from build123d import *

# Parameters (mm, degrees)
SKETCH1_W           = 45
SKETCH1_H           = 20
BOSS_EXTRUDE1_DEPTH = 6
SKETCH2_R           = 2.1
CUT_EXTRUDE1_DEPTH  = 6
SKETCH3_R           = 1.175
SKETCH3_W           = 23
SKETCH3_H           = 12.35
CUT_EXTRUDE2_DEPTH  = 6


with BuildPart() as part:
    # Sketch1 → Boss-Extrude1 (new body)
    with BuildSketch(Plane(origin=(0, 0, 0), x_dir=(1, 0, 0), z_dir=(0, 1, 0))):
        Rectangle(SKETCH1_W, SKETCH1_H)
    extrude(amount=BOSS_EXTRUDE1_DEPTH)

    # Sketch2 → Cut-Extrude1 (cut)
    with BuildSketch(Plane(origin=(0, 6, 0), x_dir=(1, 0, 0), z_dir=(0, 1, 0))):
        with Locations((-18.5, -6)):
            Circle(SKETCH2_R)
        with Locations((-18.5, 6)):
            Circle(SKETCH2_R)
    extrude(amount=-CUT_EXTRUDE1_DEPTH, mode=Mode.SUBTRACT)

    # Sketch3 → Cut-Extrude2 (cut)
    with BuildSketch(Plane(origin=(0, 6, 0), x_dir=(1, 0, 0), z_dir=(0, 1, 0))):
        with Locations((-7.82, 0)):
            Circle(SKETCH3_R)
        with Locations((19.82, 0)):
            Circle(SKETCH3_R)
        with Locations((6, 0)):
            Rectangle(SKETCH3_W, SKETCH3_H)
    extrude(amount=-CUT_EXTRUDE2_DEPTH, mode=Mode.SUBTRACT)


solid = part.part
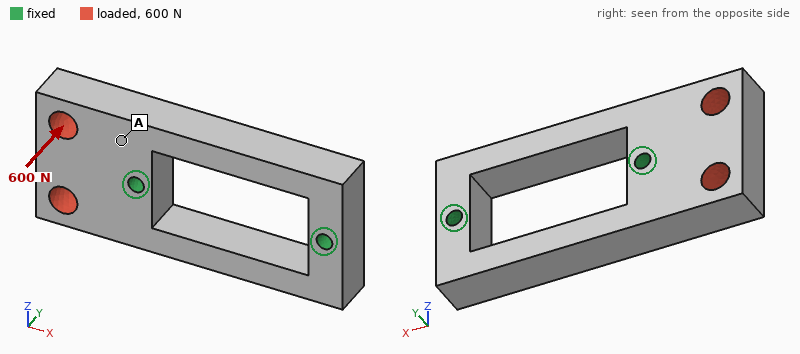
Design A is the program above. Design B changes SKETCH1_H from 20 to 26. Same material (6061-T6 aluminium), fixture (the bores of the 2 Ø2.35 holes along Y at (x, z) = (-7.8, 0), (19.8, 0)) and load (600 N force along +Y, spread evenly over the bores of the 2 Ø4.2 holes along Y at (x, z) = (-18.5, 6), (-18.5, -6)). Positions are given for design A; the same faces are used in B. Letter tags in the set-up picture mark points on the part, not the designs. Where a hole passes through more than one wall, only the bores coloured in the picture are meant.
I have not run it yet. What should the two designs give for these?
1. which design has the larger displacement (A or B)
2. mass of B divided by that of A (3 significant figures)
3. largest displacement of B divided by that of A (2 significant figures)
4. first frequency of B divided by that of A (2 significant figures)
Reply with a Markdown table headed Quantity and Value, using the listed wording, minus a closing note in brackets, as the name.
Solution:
| Quantity | Value |
|---|---|
| which design has the larger displacement | A |
| mass of B divided by that of A | 1.47 |
| largest displacement of B divided by that of A | 0.86 |
| first frequency of B divided by that of A | 0.86 |
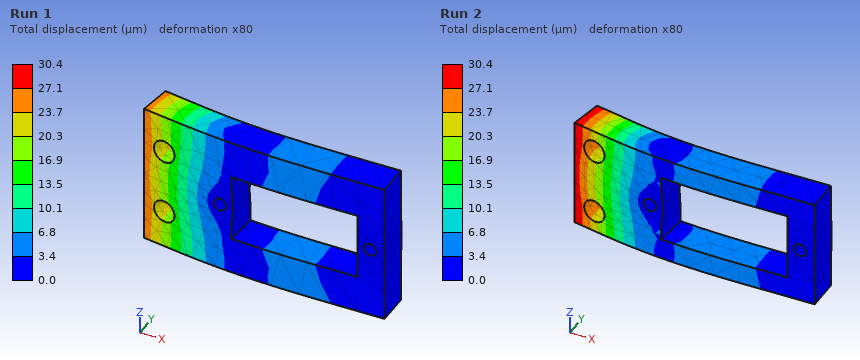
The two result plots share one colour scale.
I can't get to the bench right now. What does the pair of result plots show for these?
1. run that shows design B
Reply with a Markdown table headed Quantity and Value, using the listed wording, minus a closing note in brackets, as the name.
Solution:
| Quantity | Value |
|---|---|
| run that shows design B | Run 1 |
